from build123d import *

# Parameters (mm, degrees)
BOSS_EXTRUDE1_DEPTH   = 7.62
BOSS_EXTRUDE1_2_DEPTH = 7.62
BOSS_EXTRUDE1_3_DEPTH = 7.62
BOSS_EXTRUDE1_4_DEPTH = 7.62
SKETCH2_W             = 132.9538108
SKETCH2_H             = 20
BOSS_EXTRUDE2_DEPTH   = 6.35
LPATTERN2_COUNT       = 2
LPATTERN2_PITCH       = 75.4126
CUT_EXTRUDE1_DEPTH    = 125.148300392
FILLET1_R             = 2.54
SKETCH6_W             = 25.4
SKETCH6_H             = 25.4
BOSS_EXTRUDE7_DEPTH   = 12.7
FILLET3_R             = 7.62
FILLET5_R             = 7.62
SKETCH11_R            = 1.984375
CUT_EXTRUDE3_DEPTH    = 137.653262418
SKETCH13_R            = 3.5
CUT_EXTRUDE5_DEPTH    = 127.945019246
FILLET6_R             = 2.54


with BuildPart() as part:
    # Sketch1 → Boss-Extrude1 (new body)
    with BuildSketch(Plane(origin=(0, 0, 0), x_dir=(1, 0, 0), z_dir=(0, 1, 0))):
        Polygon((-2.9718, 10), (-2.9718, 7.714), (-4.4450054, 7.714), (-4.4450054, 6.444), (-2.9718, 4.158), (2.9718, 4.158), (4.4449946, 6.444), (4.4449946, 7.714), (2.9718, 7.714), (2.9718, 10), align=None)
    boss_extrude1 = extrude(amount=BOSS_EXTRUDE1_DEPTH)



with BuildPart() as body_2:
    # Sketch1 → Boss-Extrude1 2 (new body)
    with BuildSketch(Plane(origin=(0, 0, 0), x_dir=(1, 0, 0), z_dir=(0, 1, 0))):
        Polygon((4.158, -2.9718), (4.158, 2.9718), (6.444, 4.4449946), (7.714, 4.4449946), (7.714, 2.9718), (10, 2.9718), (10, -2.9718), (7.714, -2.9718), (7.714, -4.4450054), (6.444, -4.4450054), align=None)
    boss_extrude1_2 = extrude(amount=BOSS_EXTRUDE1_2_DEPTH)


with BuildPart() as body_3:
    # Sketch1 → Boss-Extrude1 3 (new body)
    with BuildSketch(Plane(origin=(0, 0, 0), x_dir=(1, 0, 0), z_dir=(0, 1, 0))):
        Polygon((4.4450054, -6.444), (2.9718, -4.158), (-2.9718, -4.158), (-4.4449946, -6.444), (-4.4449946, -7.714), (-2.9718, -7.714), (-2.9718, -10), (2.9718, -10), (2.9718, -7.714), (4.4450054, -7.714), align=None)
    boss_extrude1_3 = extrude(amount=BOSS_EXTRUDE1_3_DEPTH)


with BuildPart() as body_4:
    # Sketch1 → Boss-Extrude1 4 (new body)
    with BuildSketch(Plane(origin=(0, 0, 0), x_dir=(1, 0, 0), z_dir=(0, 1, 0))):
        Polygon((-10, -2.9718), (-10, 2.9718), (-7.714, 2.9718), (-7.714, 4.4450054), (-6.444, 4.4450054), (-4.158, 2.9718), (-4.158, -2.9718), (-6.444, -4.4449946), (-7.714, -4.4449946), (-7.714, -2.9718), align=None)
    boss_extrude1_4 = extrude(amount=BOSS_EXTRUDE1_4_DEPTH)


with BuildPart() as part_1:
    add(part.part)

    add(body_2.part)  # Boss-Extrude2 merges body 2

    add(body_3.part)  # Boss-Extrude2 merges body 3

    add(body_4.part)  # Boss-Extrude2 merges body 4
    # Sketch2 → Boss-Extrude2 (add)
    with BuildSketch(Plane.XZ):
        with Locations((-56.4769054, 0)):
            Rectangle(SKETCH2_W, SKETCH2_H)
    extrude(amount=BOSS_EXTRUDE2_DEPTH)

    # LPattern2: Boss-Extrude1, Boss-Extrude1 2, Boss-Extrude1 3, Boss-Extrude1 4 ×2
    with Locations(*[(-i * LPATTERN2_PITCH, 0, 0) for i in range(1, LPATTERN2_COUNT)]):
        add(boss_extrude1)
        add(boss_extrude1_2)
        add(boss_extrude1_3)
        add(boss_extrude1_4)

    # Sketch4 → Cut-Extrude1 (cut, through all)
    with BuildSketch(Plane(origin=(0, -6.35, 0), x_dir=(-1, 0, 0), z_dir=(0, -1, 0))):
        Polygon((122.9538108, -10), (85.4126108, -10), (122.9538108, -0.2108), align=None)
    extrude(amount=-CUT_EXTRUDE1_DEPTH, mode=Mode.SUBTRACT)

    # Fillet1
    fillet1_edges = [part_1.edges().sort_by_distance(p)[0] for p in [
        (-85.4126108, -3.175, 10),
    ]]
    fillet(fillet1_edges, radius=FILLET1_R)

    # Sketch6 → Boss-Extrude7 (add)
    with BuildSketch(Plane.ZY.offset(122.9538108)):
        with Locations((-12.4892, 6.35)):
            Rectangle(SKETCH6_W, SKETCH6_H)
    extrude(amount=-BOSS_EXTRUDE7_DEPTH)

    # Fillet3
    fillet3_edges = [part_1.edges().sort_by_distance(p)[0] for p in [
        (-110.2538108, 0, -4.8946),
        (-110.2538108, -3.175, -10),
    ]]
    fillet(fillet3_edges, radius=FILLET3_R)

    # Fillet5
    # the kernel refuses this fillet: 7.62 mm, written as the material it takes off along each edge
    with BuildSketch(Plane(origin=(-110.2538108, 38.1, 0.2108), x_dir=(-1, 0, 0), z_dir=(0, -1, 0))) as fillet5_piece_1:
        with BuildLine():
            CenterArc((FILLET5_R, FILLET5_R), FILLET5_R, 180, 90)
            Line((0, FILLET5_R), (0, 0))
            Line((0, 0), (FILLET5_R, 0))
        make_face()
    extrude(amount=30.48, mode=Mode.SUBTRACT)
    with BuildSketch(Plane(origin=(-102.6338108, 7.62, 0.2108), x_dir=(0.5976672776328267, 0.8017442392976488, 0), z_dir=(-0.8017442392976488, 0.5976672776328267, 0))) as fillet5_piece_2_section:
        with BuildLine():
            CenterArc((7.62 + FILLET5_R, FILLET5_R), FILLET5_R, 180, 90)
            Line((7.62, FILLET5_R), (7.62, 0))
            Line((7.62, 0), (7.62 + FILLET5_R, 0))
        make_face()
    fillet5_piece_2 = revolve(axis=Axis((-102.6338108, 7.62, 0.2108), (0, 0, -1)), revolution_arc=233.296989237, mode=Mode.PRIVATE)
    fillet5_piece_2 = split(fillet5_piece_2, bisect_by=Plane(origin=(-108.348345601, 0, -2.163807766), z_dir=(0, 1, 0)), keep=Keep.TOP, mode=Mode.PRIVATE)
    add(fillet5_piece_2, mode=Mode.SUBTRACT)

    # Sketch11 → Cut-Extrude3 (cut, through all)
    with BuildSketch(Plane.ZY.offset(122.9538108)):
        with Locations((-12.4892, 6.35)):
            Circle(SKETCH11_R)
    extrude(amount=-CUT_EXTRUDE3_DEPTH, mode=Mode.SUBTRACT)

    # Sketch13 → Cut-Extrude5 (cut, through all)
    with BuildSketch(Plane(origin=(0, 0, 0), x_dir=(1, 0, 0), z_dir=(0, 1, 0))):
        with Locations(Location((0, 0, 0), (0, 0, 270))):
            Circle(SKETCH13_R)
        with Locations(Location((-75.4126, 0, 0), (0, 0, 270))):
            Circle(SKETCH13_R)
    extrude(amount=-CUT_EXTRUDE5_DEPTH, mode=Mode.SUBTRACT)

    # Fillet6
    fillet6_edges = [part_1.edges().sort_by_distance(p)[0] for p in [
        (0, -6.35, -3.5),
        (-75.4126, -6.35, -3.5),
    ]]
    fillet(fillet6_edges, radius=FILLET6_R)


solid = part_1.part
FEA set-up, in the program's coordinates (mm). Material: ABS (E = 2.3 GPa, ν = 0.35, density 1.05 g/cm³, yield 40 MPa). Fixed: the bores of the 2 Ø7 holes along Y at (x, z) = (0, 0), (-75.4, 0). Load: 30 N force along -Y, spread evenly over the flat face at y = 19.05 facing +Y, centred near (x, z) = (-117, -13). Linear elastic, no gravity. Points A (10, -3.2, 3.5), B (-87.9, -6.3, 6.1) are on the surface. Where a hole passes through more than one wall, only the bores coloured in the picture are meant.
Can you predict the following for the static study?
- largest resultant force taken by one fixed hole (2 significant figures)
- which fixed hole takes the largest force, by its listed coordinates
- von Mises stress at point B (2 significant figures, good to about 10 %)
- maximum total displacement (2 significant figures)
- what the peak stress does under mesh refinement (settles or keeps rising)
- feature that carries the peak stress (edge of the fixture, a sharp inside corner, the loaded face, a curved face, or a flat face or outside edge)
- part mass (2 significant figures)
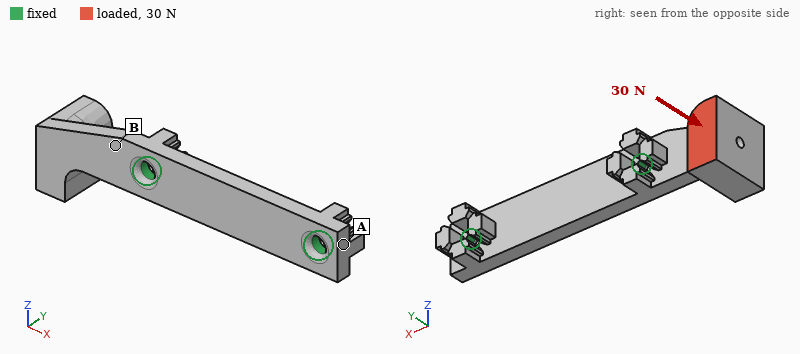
33 N
(-75.4, 0)
6.7 MPa
1.4 mm
keeps rising
edge of the fixture
26 g
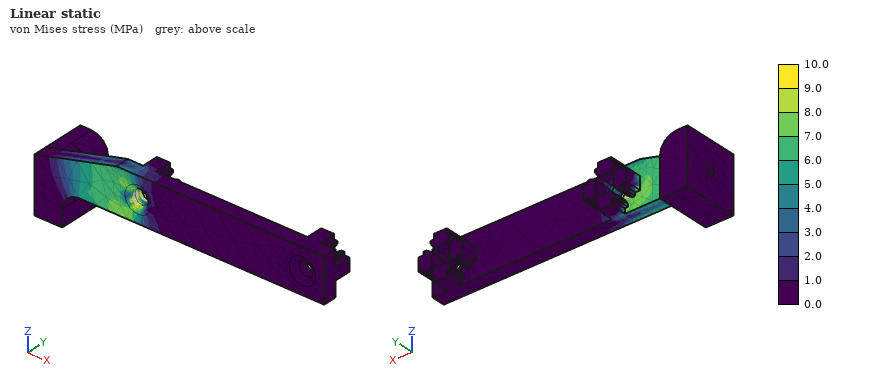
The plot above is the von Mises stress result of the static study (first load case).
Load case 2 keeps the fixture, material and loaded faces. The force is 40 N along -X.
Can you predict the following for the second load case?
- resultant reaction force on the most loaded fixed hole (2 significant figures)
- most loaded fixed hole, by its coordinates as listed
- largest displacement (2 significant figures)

45 N
(-75.4, 0)
1.4 mm
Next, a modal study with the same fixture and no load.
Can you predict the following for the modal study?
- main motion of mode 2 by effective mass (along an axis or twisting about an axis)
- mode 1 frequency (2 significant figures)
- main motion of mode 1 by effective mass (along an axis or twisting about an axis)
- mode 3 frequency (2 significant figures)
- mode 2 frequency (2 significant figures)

along Z
290 Hz
along Y
1100 Hz
540 Hz
